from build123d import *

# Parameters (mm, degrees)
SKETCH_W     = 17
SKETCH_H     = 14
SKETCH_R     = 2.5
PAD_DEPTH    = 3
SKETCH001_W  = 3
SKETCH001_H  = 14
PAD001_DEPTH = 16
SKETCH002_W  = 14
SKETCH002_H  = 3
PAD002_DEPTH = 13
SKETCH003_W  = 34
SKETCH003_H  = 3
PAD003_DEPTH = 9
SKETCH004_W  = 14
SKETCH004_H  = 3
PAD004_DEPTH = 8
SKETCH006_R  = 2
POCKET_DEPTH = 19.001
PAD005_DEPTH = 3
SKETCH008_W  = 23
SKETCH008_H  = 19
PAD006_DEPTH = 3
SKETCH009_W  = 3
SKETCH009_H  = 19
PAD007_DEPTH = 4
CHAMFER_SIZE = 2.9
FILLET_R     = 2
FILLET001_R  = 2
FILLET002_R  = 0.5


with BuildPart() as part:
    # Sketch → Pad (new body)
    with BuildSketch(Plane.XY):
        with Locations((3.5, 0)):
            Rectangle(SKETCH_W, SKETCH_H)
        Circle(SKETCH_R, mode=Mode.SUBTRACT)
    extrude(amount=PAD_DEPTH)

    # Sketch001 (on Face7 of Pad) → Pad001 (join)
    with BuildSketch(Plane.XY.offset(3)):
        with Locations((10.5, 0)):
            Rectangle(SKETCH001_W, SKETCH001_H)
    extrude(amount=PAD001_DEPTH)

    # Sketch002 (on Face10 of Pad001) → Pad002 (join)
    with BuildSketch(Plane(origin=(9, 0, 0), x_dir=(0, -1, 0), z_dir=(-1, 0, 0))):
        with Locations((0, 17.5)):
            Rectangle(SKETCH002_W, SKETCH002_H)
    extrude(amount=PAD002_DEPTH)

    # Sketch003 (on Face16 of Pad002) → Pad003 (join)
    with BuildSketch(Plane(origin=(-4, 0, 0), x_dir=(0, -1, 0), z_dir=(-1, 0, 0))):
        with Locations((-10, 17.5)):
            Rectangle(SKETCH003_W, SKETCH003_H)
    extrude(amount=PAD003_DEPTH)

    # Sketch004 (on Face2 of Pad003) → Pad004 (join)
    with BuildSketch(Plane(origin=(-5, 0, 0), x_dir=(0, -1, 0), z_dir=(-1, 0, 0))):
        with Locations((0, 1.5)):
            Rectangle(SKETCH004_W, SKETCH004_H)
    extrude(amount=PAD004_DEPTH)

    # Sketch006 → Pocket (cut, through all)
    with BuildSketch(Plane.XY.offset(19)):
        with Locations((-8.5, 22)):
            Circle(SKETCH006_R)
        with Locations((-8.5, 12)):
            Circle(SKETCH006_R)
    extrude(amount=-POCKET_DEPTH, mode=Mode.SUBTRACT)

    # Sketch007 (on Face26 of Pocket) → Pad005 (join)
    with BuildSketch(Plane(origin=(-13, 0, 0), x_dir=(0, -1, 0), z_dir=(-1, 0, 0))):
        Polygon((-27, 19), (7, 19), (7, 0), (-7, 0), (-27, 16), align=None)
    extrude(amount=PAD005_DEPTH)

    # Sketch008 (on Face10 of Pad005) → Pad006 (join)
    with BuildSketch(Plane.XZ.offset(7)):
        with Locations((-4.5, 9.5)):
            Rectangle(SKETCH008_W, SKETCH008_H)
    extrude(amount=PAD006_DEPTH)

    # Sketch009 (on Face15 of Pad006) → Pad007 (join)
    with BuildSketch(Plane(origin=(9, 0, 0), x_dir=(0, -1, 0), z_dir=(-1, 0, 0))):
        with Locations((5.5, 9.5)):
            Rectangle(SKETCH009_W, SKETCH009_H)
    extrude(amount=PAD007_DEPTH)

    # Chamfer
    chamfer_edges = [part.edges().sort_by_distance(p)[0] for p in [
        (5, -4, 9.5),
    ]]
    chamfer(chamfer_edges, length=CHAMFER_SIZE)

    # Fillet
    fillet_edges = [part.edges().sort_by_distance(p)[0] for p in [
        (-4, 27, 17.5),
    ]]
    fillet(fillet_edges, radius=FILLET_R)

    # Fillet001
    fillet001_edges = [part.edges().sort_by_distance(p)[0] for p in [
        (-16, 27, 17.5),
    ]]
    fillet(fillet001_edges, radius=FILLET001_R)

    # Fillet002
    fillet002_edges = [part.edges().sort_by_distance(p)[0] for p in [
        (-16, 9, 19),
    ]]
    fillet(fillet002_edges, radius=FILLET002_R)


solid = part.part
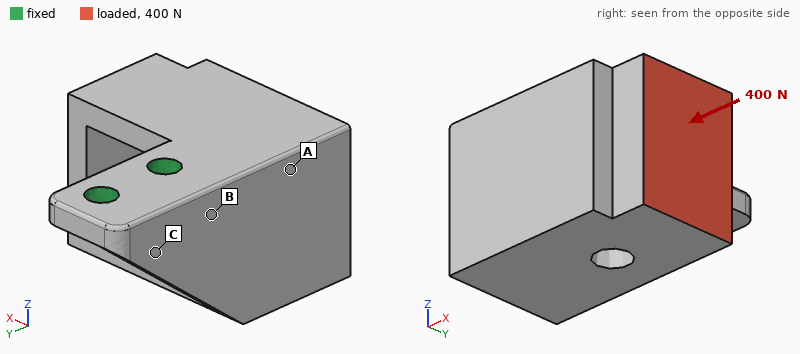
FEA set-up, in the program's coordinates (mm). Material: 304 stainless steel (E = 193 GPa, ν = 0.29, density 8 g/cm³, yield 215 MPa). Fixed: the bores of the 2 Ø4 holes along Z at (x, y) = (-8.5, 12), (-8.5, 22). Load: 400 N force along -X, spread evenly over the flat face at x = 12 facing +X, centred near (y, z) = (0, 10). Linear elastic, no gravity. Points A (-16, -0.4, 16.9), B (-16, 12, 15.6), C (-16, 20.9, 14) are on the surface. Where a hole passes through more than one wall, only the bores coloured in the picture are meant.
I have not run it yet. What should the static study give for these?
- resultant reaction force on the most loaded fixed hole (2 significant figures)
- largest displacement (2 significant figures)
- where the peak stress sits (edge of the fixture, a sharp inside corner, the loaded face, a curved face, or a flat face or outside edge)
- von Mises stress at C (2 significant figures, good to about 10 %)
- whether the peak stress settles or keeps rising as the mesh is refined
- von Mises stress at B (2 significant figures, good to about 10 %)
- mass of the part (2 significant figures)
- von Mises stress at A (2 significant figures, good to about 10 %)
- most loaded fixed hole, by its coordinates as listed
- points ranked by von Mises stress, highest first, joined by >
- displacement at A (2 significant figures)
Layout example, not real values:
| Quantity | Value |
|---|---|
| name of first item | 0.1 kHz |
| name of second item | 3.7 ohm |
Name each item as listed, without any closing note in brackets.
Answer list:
| Quantity | Value |
|---|---|
| resultant reaction force on the most loaded fixed hole | 630 N |
| largest displacement | 65 µm |
| where the peak stress sits | edge of the fixture |
| von Mises stress at C | 39 MPa |
| whether the peak stress settles or keeps rising as the mesh is refined | keeps rising |
| von Mises stress at B | 56 MPa |
| mass of the part | 47 g |
| von Mises stress at A | 18 MPa |
| most loaded fixed hole, by its coordinates as listed | (-8.5, 12) |
| points ranked by von Mises stress, highest first, joined by > | B > C > A |
| displacement at A | 15 µm |
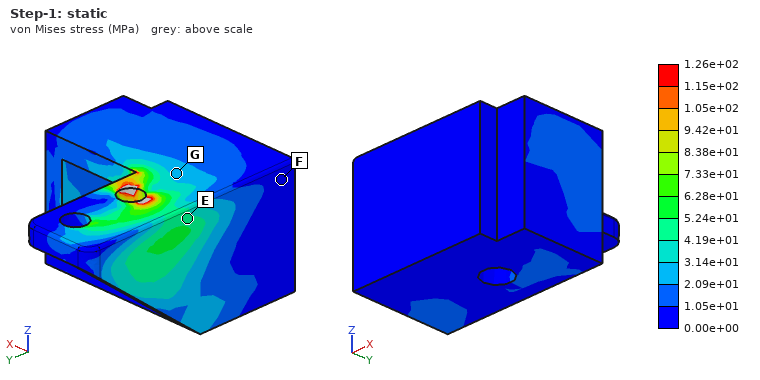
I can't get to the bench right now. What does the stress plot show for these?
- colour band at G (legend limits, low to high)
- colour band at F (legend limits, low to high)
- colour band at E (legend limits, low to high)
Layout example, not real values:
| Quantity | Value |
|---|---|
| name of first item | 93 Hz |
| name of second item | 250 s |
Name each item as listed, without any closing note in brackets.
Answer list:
| Quantity | Value |
|---|---|
| colour band at G | 2.09e+01 to 3.14e+01 MPa |
| colour band at F | 0.00e+00 to 1.05e+01 MPa |
| colour band at E | 4.19e+01 to 5.24e+01 MPa |
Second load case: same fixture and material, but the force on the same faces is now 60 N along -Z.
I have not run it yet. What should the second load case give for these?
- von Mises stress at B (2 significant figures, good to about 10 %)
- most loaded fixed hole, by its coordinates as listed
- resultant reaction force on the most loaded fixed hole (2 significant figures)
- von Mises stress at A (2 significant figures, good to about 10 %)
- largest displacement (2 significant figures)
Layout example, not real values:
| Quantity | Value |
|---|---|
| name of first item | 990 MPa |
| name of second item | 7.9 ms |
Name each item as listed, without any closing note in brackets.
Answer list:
| Quantity | Value |
|---|---|
| von Mises stress at B | 18 MPa |
| most loaded fixed hole, by its coordinates as listed | (-8.5, 12) |
| resultant reaction force on the most loaded fixed hole | 80 N |
| von Mises stress at A | 9.6 MPa |
| largest displacement | 27 µm |
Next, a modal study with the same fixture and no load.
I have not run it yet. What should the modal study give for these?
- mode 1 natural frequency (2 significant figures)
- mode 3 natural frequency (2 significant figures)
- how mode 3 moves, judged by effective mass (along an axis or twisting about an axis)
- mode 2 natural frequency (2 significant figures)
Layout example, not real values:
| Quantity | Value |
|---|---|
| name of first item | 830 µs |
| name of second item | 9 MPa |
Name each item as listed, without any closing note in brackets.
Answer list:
| Quantity | Value |
|---|---|
| mode 1 natural frequency | 1900 Hz |
| mode 3 natural frequency | 5700 Hz |
| how mode 3 moves, judged by effective mass | along Z |
| mode 2 natural frequency | 3000 Hz |
